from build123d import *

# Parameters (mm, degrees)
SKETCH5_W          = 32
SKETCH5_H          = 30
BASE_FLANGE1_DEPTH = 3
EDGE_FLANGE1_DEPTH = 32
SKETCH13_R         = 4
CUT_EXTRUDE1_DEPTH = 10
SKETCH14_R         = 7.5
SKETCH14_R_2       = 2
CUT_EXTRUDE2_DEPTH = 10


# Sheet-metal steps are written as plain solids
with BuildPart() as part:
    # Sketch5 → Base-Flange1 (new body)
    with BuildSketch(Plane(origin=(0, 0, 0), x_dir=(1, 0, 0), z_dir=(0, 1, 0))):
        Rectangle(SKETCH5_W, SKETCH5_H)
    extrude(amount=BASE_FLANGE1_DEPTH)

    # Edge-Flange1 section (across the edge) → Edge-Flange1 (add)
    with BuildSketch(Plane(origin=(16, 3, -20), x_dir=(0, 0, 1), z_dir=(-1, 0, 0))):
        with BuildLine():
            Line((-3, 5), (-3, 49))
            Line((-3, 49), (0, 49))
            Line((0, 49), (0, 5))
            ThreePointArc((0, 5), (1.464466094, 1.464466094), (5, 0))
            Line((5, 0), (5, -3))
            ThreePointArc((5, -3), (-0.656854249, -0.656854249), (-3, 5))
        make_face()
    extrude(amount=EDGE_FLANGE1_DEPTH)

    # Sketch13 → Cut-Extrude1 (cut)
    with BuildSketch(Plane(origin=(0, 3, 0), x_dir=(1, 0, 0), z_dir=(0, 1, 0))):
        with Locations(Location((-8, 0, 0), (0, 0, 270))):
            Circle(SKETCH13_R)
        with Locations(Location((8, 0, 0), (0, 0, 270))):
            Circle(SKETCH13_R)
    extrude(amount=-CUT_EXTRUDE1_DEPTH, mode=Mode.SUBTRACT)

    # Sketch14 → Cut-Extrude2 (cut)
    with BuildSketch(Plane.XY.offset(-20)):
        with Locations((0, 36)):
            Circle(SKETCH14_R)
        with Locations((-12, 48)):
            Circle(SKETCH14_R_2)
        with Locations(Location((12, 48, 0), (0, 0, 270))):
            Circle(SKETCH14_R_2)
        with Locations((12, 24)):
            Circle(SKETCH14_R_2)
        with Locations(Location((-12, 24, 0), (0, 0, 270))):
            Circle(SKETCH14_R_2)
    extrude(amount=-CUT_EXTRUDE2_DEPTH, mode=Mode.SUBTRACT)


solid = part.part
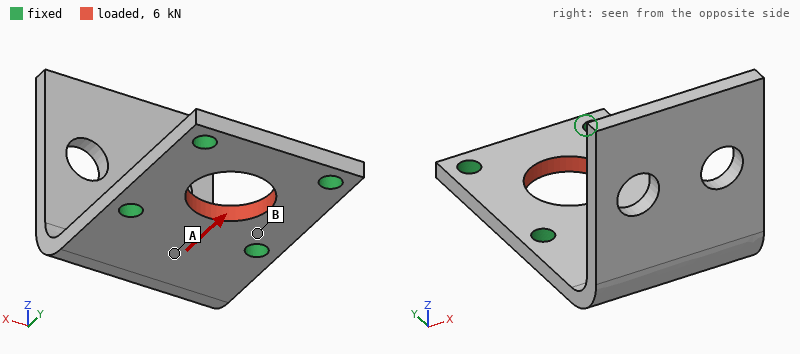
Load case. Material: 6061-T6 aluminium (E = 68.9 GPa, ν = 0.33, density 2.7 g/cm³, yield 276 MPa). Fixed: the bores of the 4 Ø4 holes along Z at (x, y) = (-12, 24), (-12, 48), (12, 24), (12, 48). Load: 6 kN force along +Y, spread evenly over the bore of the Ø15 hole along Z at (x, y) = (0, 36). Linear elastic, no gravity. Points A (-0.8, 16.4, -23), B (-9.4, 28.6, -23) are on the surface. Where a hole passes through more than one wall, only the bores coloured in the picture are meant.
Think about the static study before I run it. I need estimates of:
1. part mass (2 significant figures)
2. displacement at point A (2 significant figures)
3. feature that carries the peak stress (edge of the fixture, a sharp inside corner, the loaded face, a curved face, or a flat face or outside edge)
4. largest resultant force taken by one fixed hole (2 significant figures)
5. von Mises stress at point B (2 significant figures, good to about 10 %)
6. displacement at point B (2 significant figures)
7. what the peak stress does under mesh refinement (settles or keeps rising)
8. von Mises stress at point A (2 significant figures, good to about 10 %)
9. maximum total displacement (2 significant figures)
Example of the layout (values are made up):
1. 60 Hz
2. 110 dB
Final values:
1. 19 g
2. 4.4 µm
3. edge of the fixture
4. 1.6 kN
5. 54 MPa
6. 3.0 µm
7. keeps rising
8. 17 MPa
9. 16 µm
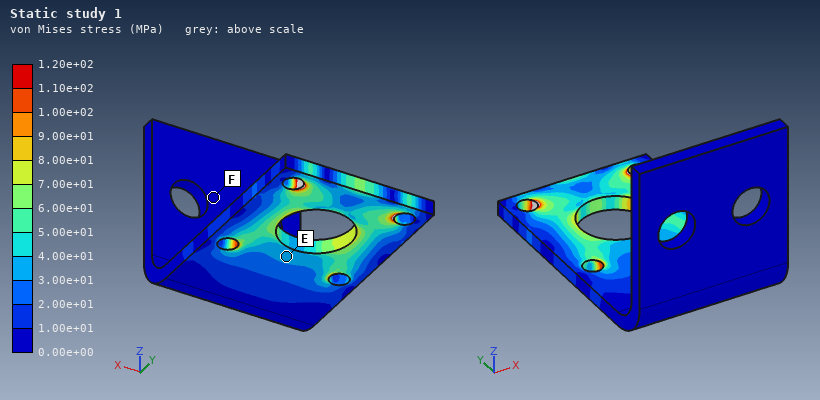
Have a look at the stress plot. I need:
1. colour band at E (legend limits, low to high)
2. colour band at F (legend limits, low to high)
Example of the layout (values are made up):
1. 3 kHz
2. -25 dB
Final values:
1. 3.00e+01 to 4.00e+01 MPa
2. 0.00e+00 to 1.00e+01 MPa
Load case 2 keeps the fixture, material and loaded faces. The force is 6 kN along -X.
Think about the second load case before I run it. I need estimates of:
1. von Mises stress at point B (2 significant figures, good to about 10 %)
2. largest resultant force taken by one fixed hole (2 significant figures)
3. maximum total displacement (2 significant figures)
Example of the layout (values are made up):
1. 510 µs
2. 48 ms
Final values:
1. 59 MPa
2. 1.6 kN
3. 15 µm
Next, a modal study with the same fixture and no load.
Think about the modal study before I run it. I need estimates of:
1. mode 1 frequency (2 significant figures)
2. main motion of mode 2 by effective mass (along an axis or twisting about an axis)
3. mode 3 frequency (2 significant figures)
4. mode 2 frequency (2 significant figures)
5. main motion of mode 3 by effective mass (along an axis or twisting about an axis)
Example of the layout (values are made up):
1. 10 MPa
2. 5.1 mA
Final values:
1. 1000 Hz
2. along X
3. 3100 Hz
4. 1900 Hz
5. along Z
